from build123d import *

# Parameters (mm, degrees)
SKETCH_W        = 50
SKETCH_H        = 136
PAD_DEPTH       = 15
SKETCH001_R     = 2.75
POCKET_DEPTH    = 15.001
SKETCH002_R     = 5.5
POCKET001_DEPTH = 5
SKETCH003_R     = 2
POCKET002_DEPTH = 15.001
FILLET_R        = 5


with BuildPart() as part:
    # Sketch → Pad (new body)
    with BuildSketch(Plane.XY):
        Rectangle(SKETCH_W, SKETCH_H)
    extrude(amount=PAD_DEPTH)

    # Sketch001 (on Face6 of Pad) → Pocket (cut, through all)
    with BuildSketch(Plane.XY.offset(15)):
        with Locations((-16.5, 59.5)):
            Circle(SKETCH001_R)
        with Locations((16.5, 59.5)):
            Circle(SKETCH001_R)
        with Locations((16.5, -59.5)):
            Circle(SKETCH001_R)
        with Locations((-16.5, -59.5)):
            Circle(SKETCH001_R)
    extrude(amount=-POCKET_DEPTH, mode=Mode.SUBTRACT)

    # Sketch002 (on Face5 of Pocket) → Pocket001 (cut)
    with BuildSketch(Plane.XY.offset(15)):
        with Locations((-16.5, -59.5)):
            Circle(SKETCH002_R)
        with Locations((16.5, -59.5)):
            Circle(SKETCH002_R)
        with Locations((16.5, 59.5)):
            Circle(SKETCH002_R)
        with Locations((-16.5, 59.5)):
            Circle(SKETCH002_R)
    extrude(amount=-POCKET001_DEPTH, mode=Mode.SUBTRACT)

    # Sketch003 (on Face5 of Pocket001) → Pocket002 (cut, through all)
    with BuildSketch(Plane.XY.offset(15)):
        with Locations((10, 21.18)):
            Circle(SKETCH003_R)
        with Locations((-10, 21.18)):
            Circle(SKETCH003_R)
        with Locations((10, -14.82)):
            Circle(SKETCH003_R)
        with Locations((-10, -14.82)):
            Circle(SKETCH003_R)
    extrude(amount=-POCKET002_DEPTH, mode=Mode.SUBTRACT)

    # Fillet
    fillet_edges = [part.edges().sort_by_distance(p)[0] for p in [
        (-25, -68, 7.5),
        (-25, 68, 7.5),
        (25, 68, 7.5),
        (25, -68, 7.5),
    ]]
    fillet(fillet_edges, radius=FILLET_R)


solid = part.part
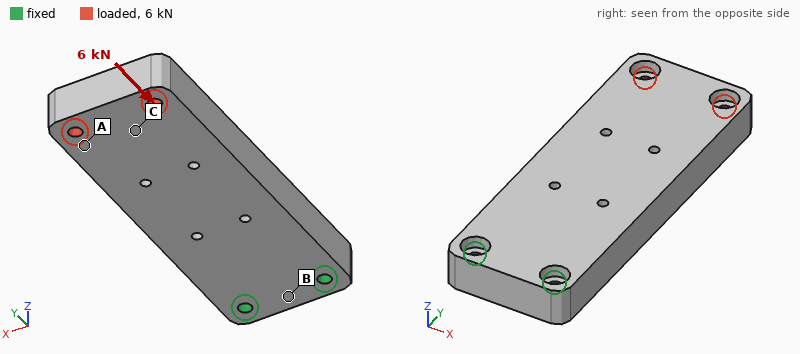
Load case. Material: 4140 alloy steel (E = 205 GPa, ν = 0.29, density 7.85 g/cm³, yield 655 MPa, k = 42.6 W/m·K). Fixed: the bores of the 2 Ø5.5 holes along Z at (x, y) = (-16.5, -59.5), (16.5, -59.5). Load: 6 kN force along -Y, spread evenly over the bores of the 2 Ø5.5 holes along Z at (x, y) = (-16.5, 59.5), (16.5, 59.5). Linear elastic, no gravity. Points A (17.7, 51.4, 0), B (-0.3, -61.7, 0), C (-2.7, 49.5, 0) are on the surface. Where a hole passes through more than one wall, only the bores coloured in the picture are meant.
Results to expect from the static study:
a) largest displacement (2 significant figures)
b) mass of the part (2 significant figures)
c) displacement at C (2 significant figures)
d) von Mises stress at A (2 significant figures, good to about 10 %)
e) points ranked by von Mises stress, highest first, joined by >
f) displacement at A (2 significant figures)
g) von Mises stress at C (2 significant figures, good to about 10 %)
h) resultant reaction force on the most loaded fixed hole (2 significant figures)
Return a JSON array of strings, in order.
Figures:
["41 µm", "770 g", "30 µm", "20 MPa", "A > C > B", "31 µm", "10 MPa", "3.0 kN"]
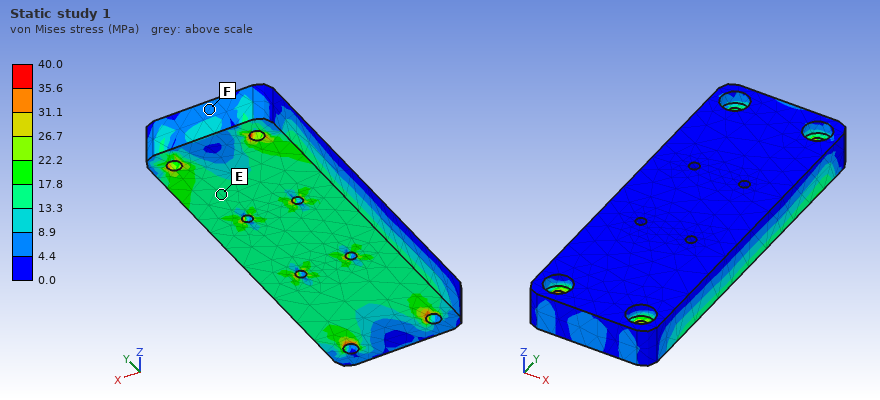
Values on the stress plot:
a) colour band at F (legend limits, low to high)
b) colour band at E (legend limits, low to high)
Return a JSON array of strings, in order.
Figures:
["4.4 to 8.9 MPa", "13.3 to 17.8 MPa"]
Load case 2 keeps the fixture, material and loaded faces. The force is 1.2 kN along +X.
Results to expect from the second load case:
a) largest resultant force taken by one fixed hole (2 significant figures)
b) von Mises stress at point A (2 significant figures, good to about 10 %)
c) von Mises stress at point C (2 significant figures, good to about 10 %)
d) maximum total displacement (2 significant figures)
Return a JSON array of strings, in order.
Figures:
["4.1 kN", "4.2 MPa", "5.2 MPa", "32 µm"]
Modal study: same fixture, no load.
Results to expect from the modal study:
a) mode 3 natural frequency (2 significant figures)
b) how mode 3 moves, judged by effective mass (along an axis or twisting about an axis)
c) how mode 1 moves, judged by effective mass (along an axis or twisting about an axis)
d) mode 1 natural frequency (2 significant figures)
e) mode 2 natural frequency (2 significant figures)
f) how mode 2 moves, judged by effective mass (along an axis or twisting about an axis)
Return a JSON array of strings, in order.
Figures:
["3400 Hz", "twisting about Y", "along Z", "640 Hz", "2200 Hz", "along X"]
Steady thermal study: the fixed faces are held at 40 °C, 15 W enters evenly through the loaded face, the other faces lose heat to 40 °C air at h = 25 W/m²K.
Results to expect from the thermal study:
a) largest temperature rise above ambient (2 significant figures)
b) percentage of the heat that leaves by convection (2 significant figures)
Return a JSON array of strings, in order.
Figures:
["39 K", "55 %"]
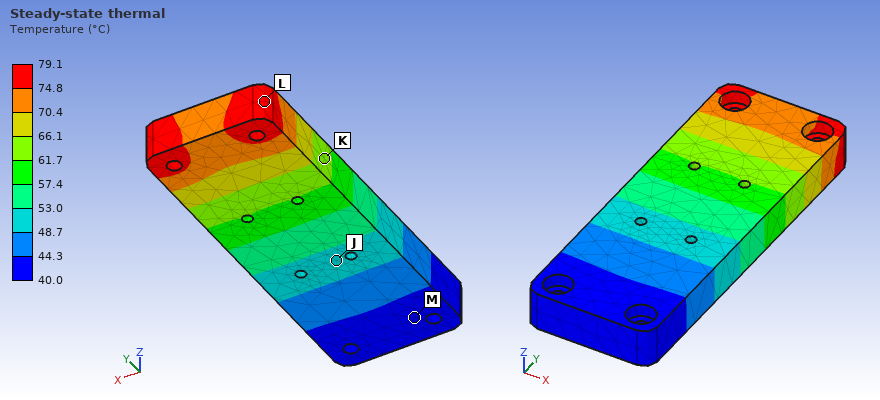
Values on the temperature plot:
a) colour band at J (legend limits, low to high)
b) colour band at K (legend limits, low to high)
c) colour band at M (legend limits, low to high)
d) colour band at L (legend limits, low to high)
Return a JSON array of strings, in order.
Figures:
["48.7 to 53.0 °C", "61.7 to 66.1 °C", "40.0 to 44.3 °C", "74.8 to 79.1 °C"]
